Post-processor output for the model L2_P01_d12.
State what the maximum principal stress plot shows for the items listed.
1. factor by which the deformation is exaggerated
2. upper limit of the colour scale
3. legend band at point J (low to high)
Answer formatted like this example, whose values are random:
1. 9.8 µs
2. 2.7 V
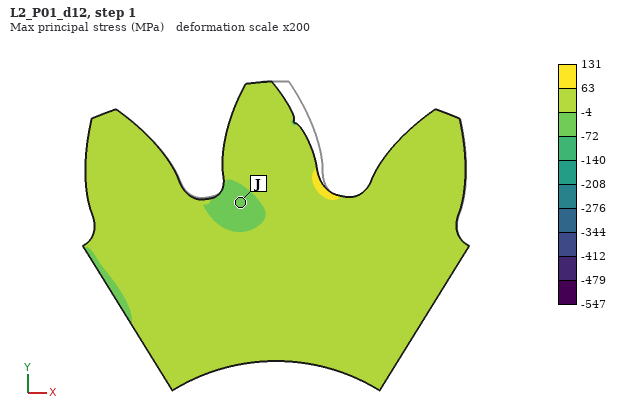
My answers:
1. 200
2. 131 MPa
3. -72 to -4 MPa
